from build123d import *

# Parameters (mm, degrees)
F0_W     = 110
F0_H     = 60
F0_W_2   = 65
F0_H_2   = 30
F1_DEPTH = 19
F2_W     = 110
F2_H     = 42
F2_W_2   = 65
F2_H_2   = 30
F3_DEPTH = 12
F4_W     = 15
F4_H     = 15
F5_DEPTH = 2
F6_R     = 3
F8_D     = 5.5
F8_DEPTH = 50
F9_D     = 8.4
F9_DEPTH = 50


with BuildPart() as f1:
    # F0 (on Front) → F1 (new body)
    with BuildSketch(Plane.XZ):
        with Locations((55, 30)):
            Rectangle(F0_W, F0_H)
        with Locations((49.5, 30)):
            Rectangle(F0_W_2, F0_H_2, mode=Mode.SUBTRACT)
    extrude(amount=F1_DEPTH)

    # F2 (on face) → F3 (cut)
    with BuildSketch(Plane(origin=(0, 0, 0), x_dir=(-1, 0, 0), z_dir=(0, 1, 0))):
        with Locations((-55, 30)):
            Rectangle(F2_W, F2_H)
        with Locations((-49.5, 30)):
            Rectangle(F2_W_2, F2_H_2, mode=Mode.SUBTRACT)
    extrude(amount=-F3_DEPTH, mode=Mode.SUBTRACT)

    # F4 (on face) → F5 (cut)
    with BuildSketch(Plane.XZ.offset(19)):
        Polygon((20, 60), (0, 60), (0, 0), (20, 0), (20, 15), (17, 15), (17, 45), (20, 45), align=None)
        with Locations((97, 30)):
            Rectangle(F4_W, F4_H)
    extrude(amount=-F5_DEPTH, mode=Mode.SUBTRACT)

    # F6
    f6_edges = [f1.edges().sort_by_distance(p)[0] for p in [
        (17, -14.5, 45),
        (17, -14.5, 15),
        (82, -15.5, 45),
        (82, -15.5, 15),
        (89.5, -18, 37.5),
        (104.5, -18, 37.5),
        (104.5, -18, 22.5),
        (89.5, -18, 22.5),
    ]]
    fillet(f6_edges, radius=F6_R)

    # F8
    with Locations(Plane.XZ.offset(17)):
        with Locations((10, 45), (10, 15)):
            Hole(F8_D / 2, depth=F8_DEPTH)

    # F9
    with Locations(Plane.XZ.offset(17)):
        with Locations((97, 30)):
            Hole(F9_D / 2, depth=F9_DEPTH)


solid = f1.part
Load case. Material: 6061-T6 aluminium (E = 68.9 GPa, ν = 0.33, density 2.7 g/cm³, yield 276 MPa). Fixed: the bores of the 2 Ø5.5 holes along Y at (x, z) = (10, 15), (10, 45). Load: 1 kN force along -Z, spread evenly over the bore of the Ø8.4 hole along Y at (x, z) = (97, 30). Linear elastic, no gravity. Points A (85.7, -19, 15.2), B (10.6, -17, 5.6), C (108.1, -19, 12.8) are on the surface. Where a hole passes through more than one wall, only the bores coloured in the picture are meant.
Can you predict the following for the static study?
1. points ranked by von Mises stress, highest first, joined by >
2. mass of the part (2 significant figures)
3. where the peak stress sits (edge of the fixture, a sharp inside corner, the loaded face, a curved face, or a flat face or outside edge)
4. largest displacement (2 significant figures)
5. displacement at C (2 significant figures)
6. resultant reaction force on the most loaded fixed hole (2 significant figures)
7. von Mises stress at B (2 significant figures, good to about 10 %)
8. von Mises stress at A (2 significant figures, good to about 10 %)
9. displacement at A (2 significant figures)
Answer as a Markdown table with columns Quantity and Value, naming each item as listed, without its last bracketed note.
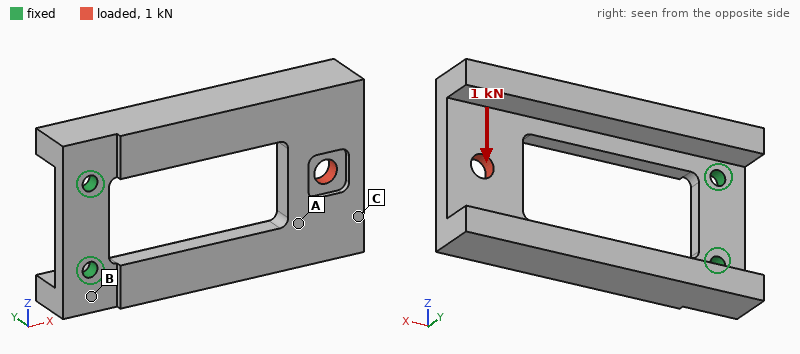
| Quantity | Value |
|---|---|
| points ranked by von Mises stress, highest first, joined by > | B > A > C |
| mass of the part | 140 g |
| where the peak stress sits | edge of the fixture |
| largest displacement | 0.28 mm |
| displacement at C | 0.25 mm |
| resultant reaction force on the most loaded fixed hole | 2.0 kN |
| von Mises stress at B | 44 MPa |
| von Mises stress at A | 24 MPa |
| displacement at A | 0.23 mm |
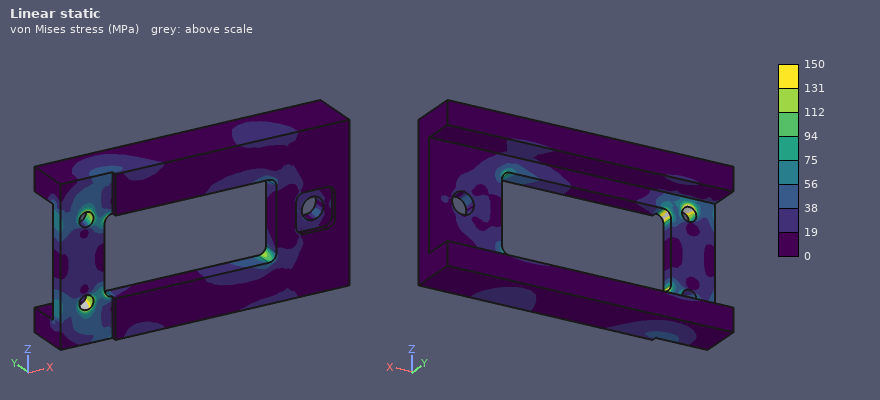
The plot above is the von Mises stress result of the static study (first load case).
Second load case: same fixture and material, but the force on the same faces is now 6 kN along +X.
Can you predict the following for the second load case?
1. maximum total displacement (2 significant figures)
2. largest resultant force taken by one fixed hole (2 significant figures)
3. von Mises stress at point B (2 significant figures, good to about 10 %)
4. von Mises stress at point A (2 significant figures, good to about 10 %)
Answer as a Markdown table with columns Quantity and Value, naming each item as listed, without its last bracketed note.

| Quantity | Value |
|---|---|
| maximum total displacement | 0.12 mm |
| largest resultant force taken by one fixed hole | 3.0 kN |
| von Mises stress at point B | 27 MPa |
| von Mises stress at point A | 41 MPa |
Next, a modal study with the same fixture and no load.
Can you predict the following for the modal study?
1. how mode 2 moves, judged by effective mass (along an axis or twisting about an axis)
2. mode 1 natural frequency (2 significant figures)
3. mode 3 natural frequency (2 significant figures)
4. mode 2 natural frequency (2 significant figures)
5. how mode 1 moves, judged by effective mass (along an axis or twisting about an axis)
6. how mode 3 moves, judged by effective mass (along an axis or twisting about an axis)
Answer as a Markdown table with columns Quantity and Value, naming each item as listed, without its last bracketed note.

| Quantity | Value |
|---|---|
| how mode 2 moves, judged by effective mass | along Z |
| mode 1 natural frequency | 570 Hz |
| mode 3 natural frequency | 1300 Hz |
| mode 2 natural frequency | 1100 Hz |
| how mode 1 moves, judged by effective mass | along Y |
| how mode 3 moves, judged by effective mass | along Z |
